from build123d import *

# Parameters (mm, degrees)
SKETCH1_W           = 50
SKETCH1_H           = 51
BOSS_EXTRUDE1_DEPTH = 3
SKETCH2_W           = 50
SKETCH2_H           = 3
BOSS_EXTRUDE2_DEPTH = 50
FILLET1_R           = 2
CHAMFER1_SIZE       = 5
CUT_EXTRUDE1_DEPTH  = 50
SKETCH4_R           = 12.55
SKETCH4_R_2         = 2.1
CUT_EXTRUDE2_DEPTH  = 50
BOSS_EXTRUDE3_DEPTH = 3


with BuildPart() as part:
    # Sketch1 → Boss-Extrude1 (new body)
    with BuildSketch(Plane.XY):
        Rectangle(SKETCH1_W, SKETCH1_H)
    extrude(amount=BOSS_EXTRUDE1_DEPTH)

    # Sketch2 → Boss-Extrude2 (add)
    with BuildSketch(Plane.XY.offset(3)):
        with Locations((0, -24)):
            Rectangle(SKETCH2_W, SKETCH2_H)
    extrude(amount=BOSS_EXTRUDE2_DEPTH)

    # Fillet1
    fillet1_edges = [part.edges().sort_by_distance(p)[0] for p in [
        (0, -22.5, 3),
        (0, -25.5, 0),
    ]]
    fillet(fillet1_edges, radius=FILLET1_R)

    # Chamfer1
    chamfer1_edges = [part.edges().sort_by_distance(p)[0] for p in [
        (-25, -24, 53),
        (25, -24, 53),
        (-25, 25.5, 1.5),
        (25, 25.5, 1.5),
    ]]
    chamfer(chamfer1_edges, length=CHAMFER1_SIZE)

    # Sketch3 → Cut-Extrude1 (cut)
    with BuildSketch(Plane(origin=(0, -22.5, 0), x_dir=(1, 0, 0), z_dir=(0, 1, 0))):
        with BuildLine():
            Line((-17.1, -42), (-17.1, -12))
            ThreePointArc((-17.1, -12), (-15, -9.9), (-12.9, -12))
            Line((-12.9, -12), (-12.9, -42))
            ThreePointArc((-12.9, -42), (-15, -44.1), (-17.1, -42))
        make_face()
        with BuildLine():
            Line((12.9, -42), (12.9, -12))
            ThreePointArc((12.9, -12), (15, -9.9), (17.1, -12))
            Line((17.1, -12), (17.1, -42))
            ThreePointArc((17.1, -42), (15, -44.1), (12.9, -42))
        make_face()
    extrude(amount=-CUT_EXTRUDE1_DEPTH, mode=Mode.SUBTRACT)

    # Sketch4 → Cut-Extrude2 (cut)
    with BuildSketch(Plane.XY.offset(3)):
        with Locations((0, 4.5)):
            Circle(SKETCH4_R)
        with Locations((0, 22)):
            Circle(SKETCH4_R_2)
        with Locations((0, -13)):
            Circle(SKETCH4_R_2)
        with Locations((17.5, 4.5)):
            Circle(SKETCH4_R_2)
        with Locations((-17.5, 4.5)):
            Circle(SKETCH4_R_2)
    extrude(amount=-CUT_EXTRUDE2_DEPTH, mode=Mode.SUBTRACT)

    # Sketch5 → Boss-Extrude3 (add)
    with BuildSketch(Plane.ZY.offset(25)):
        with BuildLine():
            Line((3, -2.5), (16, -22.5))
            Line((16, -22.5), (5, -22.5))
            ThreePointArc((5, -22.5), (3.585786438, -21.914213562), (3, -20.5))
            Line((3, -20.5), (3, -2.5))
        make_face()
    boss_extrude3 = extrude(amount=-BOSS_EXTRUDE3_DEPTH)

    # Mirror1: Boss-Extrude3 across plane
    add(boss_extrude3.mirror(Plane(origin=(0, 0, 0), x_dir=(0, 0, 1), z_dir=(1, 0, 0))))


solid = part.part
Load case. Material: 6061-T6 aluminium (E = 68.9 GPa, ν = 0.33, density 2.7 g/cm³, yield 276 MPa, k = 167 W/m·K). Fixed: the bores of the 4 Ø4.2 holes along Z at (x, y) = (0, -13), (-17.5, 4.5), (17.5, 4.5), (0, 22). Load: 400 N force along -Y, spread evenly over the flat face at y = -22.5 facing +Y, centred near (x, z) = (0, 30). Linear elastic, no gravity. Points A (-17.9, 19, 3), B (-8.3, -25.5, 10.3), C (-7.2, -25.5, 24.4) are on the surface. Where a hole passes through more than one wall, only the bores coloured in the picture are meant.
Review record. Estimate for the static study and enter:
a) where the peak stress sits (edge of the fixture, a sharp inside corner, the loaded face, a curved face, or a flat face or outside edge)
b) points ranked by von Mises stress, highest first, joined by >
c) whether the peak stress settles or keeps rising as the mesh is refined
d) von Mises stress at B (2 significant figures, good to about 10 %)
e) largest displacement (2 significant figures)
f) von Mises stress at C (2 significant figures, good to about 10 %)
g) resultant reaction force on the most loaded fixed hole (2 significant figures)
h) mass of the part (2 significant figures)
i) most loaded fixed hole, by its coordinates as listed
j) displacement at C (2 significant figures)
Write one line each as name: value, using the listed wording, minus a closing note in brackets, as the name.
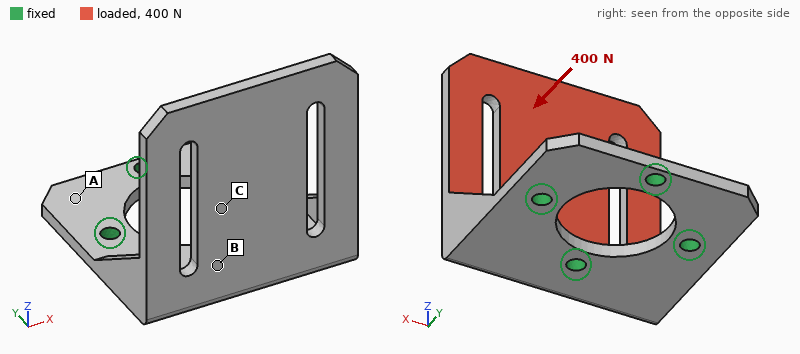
where the peak stress sits: edge of the fixture
points ranked by von Mises stress, highest first, joined by >: B > C > A
whether the peak stress settles or keeps rising as the mesh is refined: keeps rising
von Mises stress at B: 77 MPa
largest displacement: 1.0 mm
von Mises stress at C: 38 MPa
resultant reaction force on the most loaded fixed hole: 490 N
mass of the part: 36 g
most loaded fixed hole, by its coordinates as listed: (0, -13)
displacement at C: 0.34 mm
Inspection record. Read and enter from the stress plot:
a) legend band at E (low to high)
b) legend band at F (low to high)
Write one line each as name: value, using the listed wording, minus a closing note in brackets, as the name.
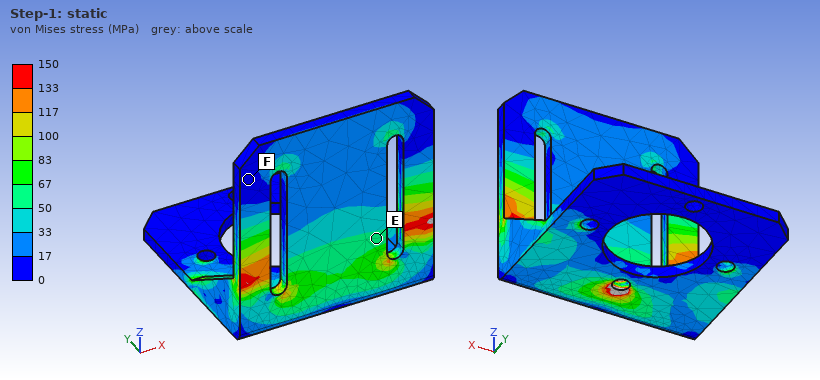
legend band at E: 50 to 67 MPa
legend band at F: 0 to 17 MPa
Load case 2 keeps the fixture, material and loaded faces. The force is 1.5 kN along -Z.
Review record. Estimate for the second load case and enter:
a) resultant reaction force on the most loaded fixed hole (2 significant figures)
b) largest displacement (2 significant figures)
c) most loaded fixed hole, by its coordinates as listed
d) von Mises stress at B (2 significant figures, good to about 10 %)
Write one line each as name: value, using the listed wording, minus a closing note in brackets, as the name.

resultant reaction force on the most loaded fixed hole: 1.7 kN
largest displacement: 0.21 mm
most loaded fixed hole, by its coordinates as listed: (0, -13)
von Mises stress at B: 34 MPa
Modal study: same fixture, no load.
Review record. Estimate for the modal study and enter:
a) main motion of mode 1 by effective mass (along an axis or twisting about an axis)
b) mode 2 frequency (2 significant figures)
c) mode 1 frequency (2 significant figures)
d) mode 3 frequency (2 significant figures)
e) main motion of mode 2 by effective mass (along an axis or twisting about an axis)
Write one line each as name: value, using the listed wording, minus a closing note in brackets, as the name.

main motion of mode 1 by effective mass: along Y
mode 2 frequency: 1300 Hz
mode 1 frequency: 970 Hz
mode 3 frequency: 2900 Hz
main motion of mode 2 by effective mass: along X
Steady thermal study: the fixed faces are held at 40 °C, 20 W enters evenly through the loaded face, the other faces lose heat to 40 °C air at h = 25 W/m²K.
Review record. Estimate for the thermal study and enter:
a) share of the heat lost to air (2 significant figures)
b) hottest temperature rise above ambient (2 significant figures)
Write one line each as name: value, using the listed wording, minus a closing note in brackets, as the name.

share of the heat lost to air: 12 %
hottest temperature rise above ambient: 32 K
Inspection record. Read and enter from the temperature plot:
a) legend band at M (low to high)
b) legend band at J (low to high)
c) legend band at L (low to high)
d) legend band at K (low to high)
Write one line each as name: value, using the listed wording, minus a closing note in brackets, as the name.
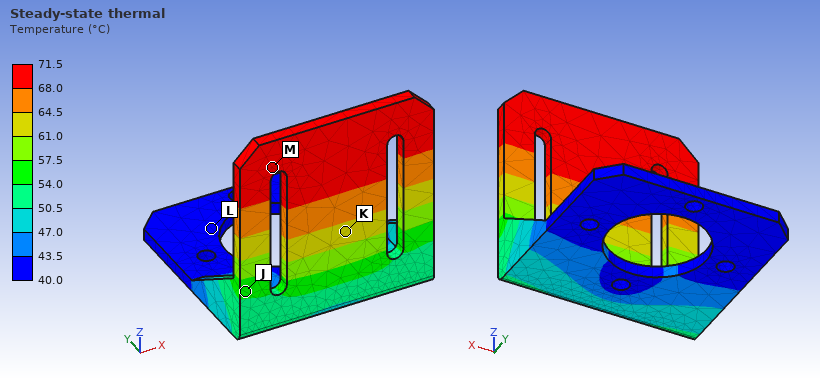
legend band at M: 68.0 to 71.5 °C
legend band at J: 54.0 to 57.5 °C
legend band at L: 40.0 to 43.5 °C
legend band at K: 61.0 to 64.5 °C
